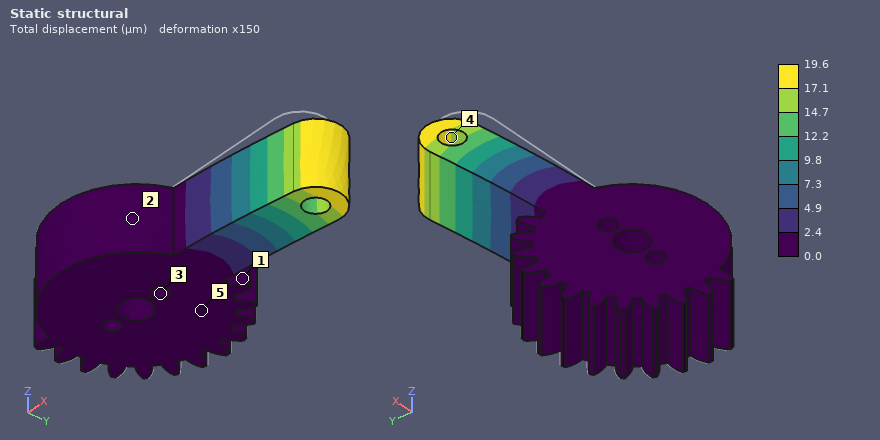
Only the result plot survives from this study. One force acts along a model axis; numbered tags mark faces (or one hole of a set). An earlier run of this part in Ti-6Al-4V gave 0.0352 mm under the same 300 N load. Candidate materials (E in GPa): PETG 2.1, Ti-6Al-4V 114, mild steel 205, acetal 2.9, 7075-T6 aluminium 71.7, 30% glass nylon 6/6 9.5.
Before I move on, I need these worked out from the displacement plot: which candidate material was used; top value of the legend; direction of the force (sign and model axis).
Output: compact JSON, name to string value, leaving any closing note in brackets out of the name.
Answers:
{"which candidate material was used": "mild steel", "top value of the legend": "19.6 µm", "direction of the force": "+Y"}
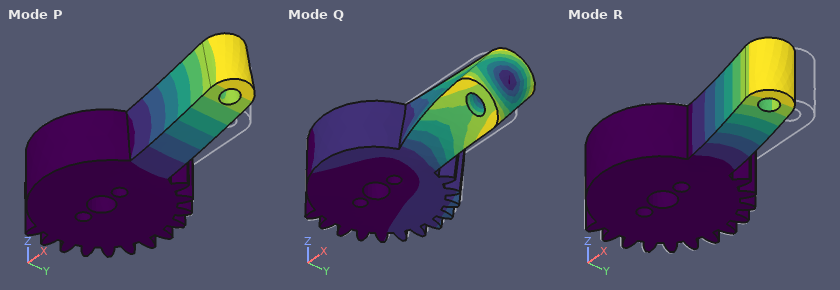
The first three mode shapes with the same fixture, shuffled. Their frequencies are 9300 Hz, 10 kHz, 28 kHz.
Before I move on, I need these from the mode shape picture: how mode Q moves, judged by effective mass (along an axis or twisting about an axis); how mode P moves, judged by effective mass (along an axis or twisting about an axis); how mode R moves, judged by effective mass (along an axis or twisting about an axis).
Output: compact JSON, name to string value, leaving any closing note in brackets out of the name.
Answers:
{"how mode Q moves, judged by effective mass": "twisting about X", "how mode P moves, judged by effective mass": "along Z", "how mode R moves, judged by effective mass": "along Y"}
